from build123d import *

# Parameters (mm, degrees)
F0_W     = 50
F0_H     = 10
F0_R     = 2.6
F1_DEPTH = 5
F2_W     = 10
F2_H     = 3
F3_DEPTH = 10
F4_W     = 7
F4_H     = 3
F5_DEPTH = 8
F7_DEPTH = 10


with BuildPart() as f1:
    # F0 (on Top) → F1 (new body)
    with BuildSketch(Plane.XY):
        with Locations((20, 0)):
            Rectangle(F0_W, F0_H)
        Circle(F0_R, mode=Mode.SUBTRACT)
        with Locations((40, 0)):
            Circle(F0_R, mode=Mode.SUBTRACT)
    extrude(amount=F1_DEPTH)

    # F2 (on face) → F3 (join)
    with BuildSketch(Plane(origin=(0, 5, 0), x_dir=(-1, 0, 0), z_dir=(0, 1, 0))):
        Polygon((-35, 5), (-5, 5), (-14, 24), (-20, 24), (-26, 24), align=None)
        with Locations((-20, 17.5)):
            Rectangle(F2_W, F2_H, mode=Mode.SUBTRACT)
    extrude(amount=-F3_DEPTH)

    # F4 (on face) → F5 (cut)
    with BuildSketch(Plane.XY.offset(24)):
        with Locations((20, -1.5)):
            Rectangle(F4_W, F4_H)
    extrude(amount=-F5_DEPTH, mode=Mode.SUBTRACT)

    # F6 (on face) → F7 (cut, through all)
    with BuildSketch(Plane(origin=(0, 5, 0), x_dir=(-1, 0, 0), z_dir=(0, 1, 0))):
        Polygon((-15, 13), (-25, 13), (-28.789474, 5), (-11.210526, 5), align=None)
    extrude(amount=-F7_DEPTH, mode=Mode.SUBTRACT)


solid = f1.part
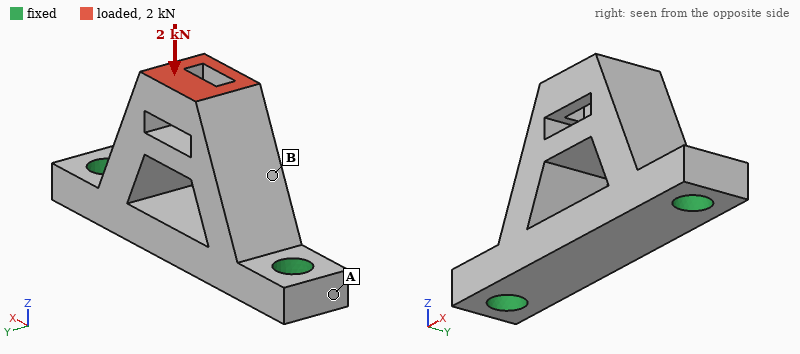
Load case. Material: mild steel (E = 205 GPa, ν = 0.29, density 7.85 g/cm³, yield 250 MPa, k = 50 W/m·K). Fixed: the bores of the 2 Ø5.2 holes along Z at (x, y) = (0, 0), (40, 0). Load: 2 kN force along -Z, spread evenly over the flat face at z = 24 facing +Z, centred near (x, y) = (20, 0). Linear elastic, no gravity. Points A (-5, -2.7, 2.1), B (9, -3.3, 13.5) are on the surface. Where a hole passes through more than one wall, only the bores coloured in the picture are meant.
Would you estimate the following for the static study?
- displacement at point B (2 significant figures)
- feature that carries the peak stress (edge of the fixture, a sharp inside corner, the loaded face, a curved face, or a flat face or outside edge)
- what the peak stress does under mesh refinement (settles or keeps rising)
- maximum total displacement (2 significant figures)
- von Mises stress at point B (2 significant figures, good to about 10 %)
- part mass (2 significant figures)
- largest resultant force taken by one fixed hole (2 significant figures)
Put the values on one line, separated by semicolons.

3.5 µm; edge of the fixture; keeps rising; 8.1 µm; 27 MPa; 37 g; 1.1 kN
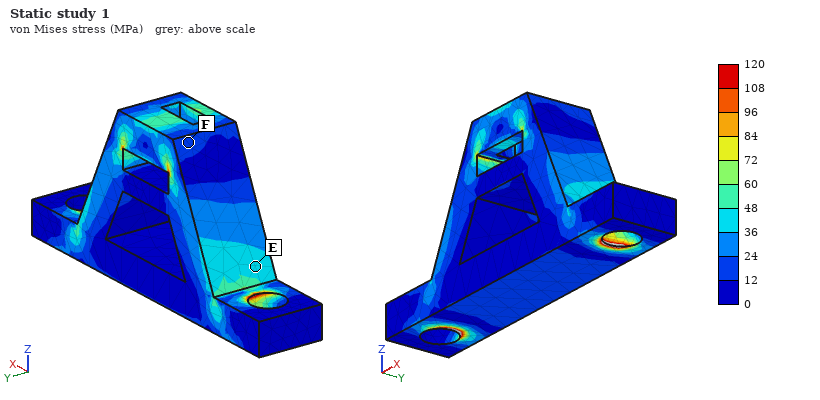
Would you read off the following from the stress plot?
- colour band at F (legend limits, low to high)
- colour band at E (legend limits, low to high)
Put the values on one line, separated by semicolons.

12 to 24 MPa; 36 to 48 MPa
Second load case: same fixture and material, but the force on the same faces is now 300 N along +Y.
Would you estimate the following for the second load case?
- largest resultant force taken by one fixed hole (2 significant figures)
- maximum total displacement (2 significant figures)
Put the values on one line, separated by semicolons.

150 N; 21 µm
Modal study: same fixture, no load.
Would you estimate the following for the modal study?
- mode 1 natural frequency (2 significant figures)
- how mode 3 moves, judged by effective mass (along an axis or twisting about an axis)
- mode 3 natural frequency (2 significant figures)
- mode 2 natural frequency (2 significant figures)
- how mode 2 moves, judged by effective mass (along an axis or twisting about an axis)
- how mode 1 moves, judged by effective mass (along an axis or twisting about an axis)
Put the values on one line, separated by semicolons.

7500 Hz; along Z; 20 kHz; 19 kHz; along X; along Y
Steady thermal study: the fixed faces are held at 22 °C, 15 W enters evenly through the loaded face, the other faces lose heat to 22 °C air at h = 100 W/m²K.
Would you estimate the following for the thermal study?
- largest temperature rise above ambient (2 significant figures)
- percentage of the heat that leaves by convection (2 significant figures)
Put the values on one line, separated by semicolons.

66 K; 41 %
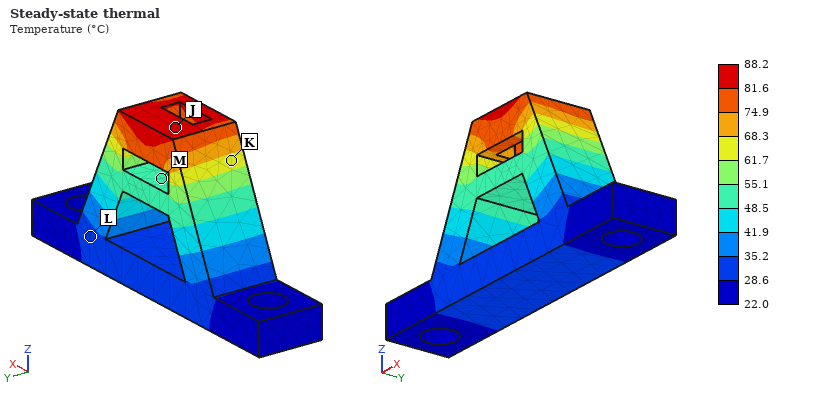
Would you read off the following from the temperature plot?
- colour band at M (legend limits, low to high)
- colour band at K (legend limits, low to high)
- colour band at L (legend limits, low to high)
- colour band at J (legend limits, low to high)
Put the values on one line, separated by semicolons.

48.5 to 55.1 °C; 61.7 to 68.3 °C; 28.6 to 35.2 °C; 81.6 to 88.2 °C
